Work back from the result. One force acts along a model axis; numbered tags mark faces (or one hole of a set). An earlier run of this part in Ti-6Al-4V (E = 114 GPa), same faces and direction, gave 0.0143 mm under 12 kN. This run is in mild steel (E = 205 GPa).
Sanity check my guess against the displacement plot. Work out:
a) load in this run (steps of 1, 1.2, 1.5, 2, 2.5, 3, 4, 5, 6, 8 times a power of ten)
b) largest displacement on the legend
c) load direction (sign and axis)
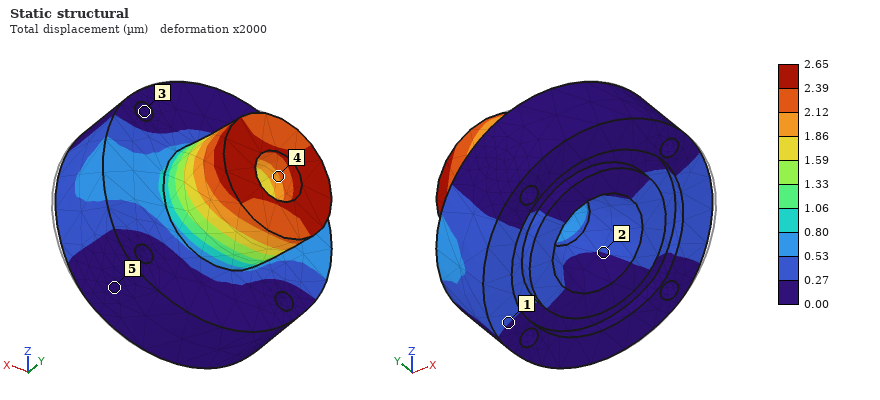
4 kN
2.65 µm
-X
